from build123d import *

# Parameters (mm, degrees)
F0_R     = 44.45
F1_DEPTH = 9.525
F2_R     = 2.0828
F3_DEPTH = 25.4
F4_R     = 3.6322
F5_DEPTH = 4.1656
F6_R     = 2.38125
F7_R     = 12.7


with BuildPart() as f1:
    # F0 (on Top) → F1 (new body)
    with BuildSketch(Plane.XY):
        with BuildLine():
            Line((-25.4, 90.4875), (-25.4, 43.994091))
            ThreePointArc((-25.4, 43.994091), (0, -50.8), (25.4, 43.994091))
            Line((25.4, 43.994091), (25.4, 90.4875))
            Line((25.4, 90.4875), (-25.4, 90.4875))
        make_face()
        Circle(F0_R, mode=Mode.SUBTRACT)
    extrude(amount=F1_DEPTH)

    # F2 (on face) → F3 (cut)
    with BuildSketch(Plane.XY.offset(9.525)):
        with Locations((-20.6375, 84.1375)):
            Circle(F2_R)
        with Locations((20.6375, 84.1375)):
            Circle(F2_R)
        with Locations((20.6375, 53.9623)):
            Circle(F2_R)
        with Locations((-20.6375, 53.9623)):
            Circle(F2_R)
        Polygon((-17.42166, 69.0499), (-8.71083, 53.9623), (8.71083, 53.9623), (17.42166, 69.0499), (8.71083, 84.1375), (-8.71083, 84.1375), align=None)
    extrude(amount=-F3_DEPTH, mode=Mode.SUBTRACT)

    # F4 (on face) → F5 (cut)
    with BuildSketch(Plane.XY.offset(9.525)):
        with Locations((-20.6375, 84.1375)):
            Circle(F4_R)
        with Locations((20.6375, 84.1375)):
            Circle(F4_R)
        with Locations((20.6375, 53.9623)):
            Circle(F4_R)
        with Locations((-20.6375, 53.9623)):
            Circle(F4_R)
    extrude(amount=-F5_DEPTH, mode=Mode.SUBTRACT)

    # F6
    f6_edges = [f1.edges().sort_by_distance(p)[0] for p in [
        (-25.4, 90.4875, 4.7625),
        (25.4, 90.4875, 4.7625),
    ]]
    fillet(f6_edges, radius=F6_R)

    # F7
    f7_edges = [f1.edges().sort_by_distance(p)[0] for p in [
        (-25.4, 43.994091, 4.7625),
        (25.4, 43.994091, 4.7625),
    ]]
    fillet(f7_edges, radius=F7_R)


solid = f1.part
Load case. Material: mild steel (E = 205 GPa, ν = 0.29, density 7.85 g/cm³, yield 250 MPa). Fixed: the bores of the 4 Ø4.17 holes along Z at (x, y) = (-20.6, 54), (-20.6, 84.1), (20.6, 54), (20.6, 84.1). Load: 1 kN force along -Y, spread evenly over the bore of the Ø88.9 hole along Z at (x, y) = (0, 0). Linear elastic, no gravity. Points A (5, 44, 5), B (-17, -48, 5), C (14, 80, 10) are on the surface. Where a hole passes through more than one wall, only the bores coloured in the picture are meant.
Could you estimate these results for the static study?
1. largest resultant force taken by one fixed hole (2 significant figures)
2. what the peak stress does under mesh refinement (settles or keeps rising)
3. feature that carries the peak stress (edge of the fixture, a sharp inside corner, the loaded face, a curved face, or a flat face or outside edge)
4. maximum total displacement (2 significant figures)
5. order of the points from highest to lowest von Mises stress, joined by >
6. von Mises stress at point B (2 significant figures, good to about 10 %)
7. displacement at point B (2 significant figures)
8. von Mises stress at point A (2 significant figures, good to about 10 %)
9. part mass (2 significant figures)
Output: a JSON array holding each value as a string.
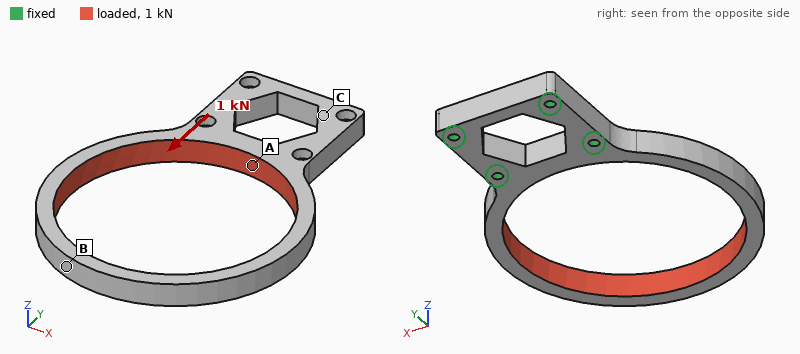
["590 N", "keeps rising", "edge of the fixture", "72 µm", "B > A > C", "26 MPa", "64 µm", "11 MPa", "240 g"]
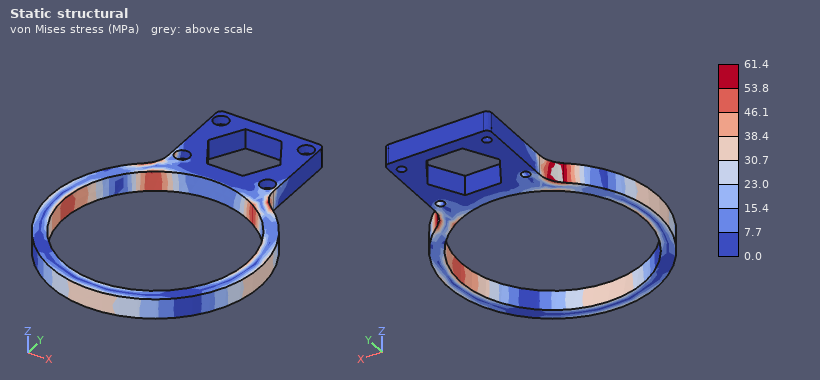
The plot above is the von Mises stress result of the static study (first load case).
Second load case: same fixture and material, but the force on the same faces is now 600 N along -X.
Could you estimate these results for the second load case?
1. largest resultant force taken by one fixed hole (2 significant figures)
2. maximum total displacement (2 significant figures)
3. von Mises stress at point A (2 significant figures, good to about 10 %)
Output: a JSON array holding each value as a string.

["670 N", "0.32 mm", "16 MPa"]
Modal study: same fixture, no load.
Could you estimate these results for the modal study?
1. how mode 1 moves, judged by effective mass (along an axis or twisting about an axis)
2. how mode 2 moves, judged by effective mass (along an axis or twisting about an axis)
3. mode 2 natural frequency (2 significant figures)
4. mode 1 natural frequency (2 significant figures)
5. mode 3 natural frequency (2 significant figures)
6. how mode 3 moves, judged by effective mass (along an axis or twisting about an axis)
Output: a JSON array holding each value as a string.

["along Z", "along X", "620 Hz", "460 Hz", "1200 Hz", "twisting about Y"]
